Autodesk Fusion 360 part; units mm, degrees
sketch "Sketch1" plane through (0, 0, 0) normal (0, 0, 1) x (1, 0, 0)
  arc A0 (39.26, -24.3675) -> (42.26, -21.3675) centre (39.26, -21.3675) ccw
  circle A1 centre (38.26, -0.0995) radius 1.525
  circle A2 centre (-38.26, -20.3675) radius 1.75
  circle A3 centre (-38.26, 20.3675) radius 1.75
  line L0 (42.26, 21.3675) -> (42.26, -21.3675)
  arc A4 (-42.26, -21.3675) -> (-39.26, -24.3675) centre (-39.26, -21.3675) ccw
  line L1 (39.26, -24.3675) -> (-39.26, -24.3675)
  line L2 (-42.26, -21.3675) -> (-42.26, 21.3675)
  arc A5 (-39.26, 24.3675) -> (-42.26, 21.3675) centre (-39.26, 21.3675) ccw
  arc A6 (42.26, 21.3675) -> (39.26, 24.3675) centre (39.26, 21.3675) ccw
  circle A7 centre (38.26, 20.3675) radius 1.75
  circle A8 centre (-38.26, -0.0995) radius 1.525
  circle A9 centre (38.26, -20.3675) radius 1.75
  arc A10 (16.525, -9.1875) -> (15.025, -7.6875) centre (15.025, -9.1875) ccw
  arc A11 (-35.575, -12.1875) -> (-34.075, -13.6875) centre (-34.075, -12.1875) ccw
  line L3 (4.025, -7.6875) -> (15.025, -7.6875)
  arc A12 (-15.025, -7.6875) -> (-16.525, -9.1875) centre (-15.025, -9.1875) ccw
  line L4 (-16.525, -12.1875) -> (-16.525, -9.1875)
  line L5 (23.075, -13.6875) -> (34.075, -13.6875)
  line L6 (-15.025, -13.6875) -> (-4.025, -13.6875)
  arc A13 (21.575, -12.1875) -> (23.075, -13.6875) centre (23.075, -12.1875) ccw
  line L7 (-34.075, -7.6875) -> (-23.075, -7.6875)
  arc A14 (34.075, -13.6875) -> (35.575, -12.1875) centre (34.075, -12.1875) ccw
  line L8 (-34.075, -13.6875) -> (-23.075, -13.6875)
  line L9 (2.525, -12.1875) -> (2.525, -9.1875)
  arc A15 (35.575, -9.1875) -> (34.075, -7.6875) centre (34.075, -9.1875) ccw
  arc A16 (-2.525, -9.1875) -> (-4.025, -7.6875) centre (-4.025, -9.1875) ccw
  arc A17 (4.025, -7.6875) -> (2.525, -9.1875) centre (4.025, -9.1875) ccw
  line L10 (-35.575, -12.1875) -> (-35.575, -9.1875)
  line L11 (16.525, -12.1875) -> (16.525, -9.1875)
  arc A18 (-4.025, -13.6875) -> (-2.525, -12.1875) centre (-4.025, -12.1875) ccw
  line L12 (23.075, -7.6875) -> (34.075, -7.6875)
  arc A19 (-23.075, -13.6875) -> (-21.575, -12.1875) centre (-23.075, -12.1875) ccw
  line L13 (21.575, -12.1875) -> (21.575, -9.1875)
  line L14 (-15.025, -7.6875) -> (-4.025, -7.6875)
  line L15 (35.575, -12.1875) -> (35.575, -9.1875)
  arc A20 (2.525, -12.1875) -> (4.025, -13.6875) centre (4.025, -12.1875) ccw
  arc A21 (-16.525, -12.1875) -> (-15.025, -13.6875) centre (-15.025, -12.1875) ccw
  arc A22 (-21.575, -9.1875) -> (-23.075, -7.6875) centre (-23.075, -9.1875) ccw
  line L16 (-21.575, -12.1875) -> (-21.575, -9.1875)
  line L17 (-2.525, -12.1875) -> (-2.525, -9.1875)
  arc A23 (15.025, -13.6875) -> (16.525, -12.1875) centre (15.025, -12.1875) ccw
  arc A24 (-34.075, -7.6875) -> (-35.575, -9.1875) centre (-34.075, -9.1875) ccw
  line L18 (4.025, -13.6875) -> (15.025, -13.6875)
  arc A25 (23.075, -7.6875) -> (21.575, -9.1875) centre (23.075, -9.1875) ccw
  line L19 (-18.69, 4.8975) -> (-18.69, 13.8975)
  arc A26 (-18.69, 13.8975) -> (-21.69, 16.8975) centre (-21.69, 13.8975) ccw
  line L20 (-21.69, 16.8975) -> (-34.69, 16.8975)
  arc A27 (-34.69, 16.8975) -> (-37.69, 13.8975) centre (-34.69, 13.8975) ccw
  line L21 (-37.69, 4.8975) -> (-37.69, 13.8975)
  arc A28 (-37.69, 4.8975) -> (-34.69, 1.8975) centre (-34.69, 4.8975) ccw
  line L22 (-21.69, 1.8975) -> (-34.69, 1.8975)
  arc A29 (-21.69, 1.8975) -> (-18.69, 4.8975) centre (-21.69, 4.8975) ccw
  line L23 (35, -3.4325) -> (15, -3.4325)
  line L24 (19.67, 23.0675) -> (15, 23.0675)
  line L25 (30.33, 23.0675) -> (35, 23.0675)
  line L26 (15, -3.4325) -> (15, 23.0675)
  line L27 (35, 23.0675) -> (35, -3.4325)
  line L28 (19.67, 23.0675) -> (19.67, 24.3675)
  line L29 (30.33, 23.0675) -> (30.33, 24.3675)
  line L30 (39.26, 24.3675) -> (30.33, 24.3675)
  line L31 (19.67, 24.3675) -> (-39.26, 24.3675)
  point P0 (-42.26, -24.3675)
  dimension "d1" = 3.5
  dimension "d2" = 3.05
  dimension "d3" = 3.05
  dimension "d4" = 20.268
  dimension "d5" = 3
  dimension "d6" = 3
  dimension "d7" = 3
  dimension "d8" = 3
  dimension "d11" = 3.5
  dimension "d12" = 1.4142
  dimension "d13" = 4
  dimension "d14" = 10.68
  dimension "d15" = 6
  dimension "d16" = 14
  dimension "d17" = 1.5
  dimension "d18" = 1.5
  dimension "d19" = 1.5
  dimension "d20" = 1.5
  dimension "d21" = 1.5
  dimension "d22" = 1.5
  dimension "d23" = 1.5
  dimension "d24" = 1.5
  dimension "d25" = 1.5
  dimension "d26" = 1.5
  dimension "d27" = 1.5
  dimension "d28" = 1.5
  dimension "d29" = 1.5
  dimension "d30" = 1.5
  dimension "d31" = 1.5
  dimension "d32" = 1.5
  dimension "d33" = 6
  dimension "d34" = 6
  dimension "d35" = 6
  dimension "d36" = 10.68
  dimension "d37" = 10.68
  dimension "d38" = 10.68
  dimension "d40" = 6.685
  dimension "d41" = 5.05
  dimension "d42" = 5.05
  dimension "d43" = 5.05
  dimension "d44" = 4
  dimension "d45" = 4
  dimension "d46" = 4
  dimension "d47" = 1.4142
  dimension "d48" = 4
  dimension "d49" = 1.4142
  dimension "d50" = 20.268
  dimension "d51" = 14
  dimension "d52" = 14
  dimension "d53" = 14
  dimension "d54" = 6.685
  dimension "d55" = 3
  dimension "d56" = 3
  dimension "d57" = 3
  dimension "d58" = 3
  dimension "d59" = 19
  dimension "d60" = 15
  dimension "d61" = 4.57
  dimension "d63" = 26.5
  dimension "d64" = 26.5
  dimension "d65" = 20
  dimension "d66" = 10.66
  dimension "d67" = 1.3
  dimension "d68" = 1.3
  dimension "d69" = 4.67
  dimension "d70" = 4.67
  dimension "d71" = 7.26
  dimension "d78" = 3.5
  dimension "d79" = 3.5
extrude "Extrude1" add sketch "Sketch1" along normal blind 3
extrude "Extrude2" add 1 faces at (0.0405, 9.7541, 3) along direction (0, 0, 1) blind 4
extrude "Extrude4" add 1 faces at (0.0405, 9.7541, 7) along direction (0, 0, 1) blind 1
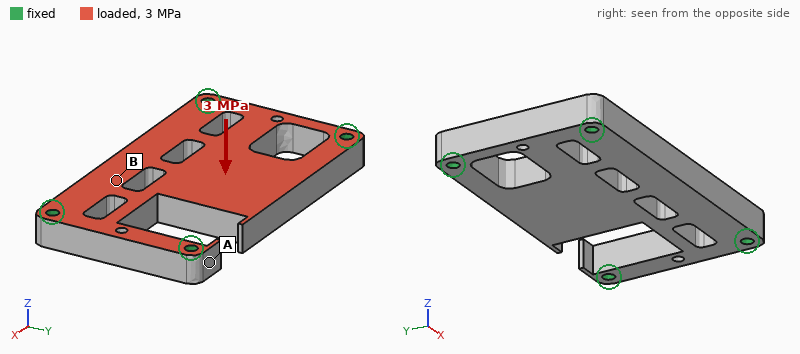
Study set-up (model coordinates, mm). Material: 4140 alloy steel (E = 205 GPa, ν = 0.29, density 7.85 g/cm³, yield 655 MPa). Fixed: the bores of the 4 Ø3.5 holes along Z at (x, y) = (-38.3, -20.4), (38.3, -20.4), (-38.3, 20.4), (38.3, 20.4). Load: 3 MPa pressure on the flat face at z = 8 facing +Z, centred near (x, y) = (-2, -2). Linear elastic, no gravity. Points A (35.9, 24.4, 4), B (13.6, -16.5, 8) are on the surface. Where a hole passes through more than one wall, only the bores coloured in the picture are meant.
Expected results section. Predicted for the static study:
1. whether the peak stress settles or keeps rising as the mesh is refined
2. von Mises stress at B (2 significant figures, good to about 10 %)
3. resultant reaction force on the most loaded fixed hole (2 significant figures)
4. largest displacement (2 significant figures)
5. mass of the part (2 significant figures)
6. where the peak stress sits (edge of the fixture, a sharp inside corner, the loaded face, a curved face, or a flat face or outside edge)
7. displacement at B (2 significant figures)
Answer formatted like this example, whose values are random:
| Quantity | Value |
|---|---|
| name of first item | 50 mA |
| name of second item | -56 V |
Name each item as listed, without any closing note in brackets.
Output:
| Quantity | Value |
|---|---|
| whether the peak stress settles or keeps rising as the mesh is refined | keeps rising |
| von Mises stress at B | 94 MPa |
| resultant reaction force on the most loaded fixed hole | 3.0 kN |
| largest displacement | 0.19 mm |
| mass of the part | 180 g |
| where the peak stress sits | edge of the fixture |
| displacement at B | 0.053 mm |
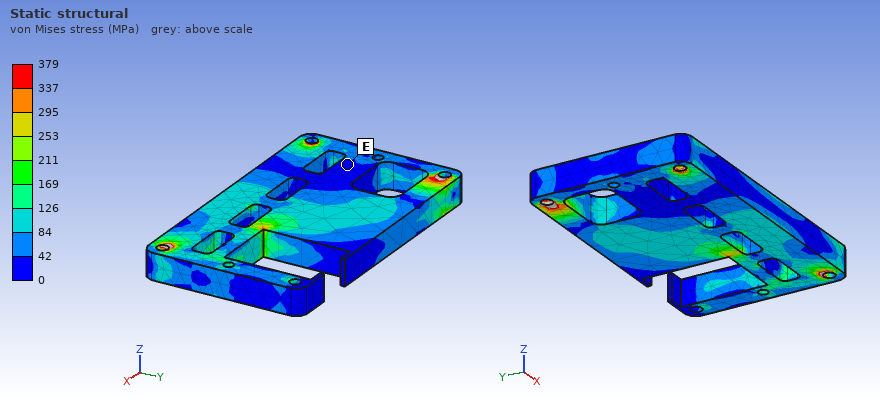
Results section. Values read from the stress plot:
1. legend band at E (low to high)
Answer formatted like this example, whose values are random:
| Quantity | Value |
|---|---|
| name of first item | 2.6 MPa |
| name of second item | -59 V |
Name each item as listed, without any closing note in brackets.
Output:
| Quantity | Value |
|---|---|
| legend band at E | 0 to 42 MPa |
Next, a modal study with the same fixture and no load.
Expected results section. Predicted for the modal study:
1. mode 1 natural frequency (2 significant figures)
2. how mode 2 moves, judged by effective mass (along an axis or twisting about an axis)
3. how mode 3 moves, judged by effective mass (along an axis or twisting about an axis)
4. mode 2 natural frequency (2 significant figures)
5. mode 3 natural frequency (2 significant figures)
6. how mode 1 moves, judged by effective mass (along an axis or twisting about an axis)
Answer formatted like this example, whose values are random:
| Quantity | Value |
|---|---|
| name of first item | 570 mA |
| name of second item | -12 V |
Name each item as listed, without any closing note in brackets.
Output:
| Quantity | Value |
|---|---|
| mode 1 natural frequency | 3500 Hz |
| how mode 2 moves, judged by effective mass | along Z |
| how mode 3 moves, judged by effective mass | along Y |
| mode 2 natural frequency | 6800 Hz |
| mode 3 natural frequency | 7900 Hz |
| how mode 1 moves, judged by effective mass | along Z |
